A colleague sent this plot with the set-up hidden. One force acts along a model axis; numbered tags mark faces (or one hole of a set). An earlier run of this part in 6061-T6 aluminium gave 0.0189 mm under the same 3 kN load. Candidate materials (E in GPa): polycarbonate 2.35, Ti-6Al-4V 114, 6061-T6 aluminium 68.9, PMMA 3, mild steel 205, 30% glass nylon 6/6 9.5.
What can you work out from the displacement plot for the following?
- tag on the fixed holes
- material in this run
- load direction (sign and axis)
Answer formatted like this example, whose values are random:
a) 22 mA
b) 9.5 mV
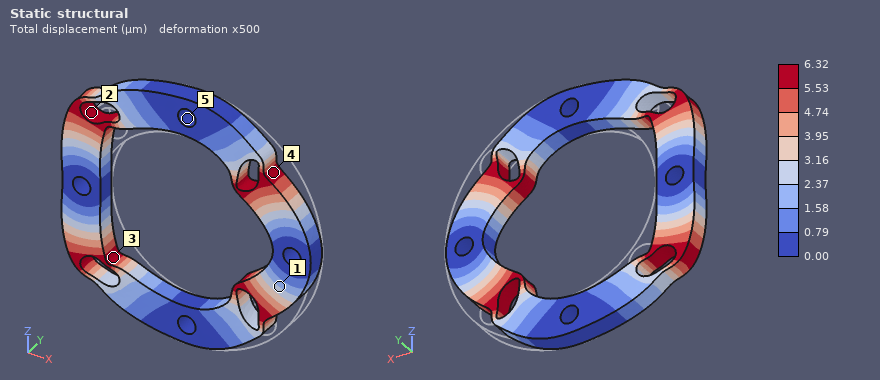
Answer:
a) 5
b) mild steel
c) -X
